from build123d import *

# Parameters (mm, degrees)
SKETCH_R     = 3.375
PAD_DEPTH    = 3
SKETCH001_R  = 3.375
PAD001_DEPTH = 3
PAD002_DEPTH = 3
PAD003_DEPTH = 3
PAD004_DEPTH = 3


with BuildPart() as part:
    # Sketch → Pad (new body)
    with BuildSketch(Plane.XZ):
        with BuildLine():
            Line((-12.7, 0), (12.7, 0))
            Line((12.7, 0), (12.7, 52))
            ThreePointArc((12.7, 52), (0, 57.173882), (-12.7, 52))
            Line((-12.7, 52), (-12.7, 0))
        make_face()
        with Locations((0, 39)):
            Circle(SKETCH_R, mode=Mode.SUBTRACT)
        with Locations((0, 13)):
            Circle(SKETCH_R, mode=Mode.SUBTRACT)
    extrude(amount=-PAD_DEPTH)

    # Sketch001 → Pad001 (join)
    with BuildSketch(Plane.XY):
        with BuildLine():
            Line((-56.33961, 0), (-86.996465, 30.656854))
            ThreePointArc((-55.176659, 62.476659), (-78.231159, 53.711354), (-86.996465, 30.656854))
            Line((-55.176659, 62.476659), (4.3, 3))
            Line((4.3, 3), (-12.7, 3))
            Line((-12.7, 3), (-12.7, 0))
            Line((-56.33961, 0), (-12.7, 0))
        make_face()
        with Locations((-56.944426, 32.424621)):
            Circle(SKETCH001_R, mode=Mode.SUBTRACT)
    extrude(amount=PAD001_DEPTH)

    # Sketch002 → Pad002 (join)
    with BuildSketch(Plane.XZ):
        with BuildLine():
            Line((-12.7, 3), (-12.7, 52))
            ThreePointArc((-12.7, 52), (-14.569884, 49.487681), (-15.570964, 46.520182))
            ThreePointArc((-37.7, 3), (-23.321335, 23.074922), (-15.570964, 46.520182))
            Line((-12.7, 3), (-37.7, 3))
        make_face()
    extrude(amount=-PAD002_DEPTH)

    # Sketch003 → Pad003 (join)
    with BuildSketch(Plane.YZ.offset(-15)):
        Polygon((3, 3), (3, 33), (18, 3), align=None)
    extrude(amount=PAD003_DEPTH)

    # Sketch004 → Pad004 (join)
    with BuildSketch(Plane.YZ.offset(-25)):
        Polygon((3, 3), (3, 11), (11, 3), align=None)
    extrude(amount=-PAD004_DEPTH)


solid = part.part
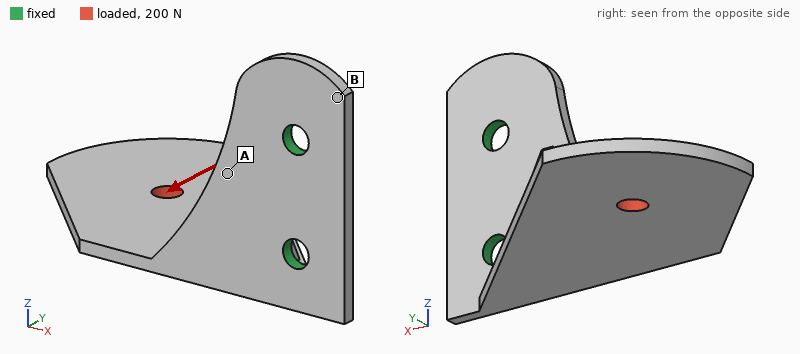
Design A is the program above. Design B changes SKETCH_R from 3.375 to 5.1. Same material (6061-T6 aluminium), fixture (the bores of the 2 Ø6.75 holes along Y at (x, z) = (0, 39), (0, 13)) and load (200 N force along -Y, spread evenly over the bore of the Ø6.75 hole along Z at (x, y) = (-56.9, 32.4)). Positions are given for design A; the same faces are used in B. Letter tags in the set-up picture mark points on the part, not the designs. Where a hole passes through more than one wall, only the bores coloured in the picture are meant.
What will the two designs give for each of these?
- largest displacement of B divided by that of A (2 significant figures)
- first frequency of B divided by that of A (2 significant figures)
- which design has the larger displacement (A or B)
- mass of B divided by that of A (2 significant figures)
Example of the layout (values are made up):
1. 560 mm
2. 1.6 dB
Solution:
1. 0.72
2. 1.0
3. A
4. 0.98
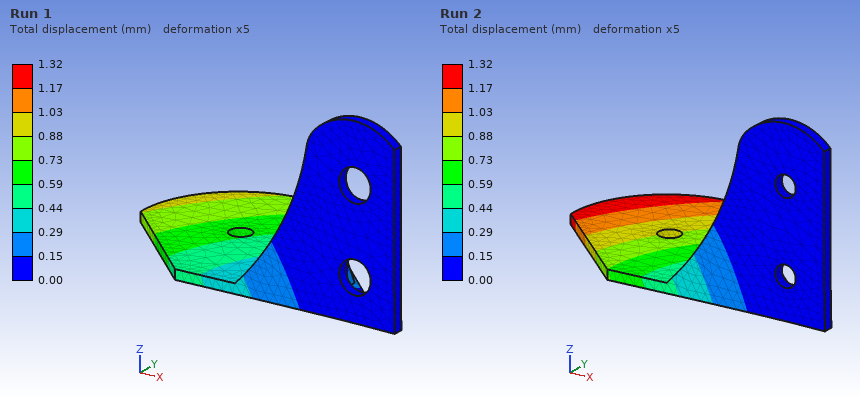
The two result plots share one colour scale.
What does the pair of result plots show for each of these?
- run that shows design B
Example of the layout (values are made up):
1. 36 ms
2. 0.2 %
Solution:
1. Run 1
